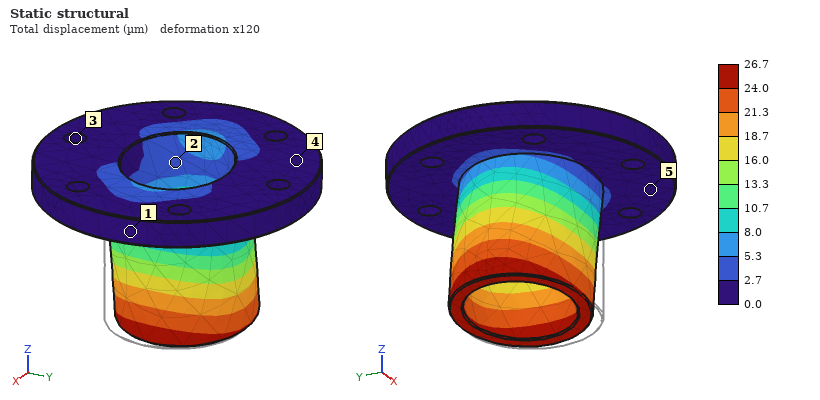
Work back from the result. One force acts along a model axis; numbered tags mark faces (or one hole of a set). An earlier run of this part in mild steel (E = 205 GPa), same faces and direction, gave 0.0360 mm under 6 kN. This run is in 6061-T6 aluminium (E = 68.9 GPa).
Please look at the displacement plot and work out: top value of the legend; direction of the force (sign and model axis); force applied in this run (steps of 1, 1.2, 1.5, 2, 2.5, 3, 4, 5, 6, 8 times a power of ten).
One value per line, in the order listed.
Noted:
26.7 µm
-X
1.5 kN
